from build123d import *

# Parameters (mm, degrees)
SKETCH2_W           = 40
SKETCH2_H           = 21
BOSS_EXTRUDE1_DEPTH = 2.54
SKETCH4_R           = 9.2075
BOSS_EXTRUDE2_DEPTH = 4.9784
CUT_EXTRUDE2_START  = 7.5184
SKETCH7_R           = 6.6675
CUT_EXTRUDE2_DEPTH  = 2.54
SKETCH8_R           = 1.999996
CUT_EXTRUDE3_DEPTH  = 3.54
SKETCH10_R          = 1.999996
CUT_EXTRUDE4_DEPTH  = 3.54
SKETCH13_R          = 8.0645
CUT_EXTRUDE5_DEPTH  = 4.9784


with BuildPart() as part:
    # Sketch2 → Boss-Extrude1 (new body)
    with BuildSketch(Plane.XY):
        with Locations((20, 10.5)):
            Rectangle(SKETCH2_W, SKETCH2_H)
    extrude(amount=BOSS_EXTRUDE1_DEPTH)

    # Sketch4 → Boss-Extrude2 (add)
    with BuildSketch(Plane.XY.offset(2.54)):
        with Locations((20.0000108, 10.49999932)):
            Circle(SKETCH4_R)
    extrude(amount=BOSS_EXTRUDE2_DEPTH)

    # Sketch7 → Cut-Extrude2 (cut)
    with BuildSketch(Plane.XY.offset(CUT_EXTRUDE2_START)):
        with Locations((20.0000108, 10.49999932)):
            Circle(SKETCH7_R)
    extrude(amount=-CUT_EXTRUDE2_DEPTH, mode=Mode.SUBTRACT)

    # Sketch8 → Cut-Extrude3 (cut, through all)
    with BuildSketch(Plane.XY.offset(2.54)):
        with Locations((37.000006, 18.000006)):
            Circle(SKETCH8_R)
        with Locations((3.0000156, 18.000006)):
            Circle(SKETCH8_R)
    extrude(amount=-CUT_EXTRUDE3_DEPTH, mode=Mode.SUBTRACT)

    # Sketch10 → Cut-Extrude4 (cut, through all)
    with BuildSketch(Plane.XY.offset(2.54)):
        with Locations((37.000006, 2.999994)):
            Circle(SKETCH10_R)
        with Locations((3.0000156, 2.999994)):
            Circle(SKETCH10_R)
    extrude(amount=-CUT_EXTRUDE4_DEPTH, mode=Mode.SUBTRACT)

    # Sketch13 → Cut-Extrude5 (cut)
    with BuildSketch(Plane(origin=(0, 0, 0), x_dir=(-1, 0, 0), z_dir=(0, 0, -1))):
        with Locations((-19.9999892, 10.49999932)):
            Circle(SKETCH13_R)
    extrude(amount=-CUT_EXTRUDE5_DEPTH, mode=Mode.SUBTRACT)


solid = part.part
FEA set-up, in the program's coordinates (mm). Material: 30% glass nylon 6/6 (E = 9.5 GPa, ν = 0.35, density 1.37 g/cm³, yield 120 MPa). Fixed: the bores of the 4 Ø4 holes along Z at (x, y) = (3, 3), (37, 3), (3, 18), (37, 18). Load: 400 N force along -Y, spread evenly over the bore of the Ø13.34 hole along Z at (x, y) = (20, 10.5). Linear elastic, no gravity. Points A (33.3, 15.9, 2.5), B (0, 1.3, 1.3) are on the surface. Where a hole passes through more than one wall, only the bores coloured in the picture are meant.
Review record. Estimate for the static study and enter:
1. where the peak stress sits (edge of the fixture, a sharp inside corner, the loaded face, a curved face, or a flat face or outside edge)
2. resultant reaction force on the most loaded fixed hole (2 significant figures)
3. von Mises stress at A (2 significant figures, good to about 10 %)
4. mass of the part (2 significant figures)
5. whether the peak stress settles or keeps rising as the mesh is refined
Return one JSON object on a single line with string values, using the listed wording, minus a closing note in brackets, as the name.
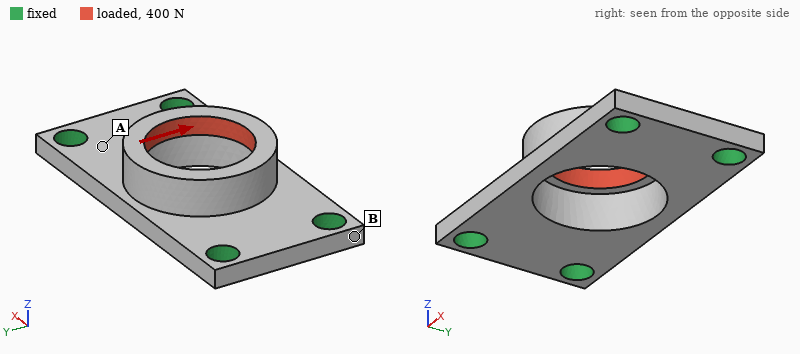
{"where the peak stress sits": "edge of the fixture", "resultant reaction force on the most loaded fixed hole": "150 N", "von Mises stress at A": "22 MPa", "mass of the part": "2.7 g", "whether the peak stress settles or keeps rising as the mesh is refined": "keeps rising"}
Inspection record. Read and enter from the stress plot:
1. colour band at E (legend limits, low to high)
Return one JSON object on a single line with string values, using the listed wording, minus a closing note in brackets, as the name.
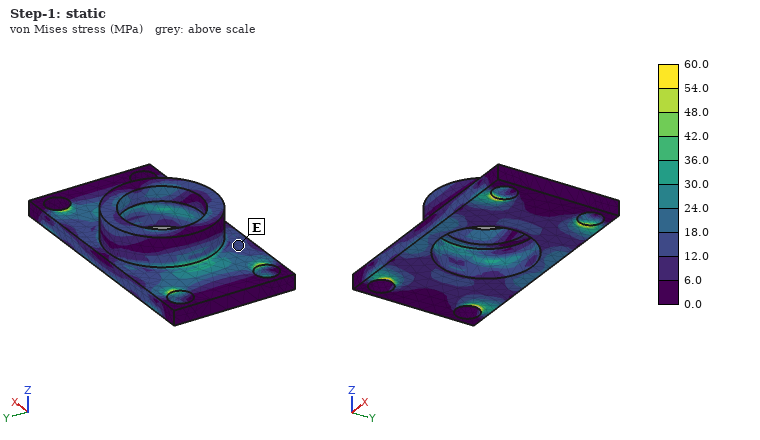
{"colour band at E": "12.0 to 18.0 MPa"}
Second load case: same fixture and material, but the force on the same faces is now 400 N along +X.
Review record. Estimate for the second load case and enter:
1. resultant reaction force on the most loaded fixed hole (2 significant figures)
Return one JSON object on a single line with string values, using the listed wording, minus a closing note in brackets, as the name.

{"resultant reaction force on the most loaded fixed hole": "110 N"}
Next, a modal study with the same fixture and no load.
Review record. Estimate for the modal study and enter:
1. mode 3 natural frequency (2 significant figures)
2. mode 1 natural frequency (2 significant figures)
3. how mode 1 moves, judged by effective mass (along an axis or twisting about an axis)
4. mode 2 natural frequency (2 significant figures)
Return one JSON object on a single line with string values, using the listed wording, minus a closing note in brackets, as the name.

{"mode 3 natural frequency": "14 kHz", "mode 1 natural frequency": "7700 Hz", "how mode 1 moves, judged by effective mass": "along Z", "mode 2 natural frequency": "8100 Hz"}
